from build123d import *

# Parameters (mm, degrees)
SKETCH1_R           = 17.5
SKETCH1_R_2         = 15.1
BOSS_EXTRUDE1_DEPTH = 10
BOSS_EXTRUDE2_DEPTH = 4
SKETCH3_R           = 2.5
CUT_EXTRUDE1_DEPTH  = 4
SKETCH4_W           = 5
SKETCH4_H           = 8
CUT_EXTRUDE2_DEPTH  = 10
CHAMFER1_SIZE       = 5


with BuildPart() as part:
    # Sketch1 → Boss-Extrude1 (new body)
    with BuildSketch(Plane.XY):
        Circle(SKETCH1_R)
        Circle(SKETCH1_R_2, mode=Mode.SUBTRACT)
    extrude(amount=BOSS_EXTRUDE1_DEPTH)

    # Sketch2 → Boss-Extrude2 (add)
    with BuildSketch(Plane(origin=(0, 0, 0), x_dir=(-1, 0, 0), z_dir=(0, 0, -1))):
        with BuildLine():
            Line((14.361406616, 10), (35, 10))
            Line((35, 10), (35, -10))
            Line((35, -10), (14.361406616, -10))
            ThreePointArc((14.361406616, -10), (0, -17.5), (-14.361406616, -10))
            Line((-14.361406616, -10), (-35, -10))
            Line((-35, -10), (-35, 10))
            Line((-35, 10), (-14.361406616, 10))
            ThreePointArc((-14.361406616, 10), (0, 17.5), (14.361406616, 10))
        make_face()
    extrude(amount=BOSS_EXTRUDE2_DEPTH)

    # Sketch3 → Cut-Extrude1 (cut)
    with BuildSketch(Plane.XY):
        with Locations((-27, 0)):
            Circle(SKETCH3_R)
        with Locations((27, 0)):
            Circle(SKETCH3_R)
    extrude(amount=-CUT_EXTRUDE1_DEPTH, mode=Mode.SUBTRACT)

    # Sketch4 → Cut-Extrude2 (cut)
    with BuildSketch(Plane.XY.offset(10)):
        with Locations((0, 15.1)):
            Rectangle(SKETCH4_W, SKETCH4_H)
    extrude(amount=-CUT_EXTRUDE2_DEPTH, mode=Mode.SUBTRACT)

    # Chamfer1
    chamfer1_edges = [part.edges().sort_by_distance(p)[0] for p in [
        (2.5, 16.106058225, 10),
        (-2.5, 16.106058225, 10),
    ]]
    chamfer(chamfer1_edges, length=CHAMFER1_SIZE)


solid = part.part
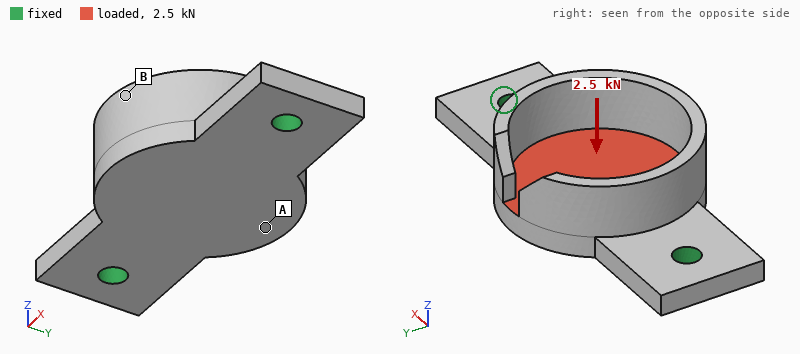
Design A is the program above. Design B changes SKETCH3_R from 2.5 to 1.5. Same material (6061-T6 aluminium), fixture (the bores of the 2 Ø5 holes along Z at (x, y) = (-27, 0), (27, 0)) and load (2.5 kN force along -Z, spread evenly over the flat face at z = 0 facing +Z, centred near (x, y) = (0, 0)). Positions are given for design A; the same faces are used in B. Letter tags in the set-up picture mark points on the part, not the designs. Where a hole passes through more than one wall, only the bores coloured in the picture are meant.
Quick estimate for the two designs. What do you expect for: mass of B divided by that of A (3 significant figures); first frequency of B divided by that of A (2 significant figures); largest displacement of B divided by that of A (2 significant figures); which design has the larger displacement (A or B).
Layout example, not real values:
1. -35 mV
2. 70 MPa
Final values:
1. 1.01
2. 0.89
3. 1.2
4. B
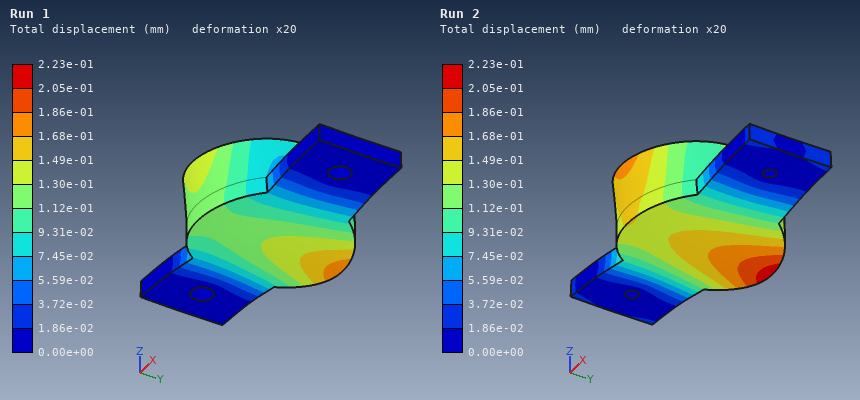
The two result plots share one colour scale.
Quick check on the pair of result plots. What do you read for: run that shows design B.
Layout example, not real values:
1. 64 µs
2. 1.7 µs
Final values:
1. Run 2
